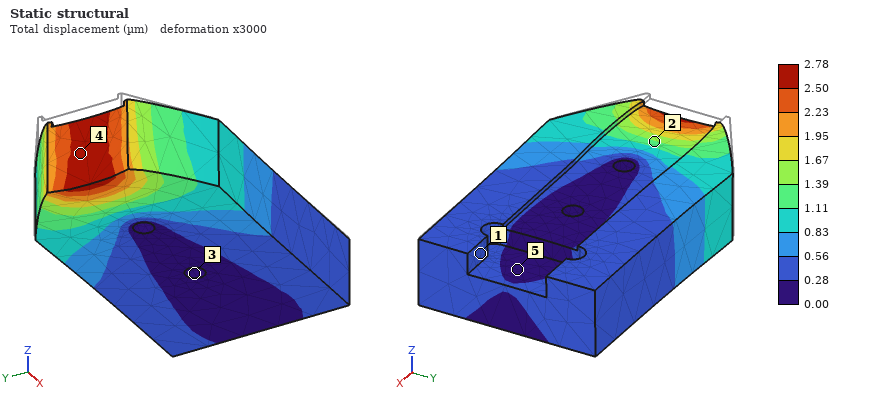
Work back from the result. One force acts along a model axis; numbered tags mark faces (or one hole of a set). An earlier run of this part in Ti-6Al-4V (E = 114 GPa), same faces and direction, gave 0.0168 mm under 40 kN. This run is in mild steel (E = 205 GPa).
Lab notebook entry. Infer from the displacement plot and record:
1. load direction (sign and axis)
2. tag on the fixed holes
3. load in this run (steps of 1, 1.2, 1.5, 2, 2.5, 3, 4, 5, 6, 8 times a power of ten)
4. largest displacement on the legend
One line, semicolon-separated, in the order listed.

+X; 3; 12 kN; 2.78 µm
